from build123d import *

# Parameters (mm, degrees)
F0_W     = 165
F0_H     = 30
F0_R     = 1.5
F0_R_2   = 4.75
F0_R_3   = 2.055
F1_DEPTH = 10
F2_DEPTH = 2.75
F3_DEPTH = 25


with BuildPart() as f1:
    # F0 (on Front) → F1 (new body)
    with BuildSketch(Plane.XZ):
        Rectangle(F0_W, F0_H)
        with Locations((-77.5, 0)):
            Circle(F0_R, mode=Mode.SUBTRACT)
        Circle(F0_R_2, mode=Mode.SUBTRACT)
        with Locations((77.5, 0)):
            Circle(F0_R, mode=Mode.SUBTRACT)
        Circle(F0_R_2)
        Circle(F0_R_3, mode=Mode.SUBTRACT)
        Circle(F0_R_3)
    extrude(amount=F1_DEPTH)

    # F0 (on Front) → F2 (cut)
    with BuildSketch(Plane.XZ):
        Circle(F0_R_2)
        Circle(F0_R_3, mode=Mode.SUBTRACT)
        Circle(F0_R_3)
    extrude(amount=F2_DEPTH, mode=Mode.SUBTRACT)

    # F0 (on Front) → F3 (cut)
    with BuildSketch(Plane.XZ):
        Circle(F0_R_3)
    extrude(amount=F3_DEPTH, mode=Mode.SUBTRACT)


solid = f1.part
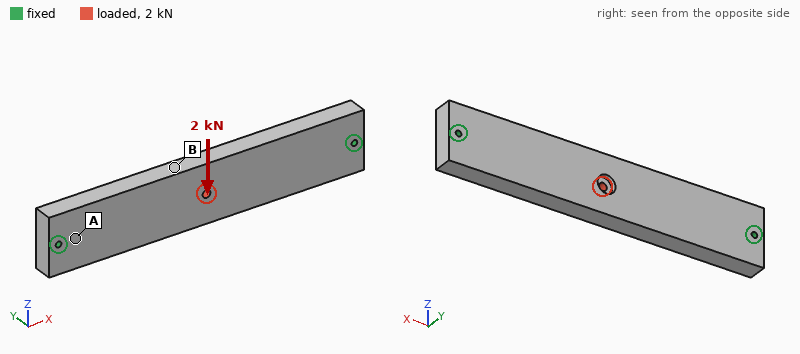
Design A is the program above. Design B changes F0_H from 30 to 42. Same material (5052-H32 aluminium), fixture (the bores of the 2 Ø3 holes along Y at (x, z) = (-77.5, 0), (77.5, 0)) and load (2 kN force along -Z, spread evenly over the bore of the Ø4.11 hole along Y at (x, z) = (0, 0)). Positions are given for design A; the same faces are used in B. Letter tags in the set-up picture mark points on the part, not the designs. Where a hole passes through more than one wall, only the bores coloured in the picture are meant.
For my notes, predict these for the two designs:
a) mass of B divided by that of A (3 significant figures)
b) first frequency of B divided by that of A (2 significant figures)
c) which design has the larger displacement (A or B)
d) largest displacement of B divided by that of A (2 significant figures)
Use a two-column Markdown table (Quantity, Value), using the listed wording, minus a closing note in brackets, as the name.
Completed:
| Quantity | Value |
|---|---|
| mass of B divided by that of A | 1.40 |
| first frequency of B divided by that of A | 0.93 |
| which design has the larger displacement | A |
| largest displacement of B divided by that of A | 0.47 |
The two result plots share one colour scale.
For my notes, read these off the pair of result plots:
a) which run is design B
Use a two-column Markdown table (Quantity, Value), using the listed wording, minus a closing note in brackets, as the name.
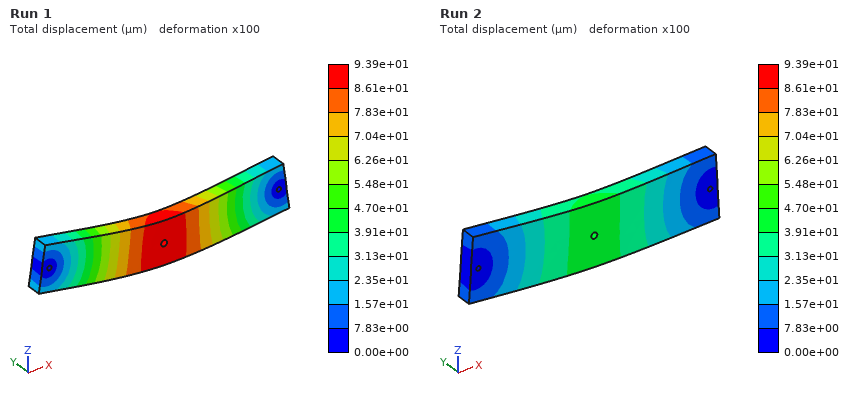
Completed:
| Quantity | Value |
|---|---|
| which run is design B | Run 2 |
